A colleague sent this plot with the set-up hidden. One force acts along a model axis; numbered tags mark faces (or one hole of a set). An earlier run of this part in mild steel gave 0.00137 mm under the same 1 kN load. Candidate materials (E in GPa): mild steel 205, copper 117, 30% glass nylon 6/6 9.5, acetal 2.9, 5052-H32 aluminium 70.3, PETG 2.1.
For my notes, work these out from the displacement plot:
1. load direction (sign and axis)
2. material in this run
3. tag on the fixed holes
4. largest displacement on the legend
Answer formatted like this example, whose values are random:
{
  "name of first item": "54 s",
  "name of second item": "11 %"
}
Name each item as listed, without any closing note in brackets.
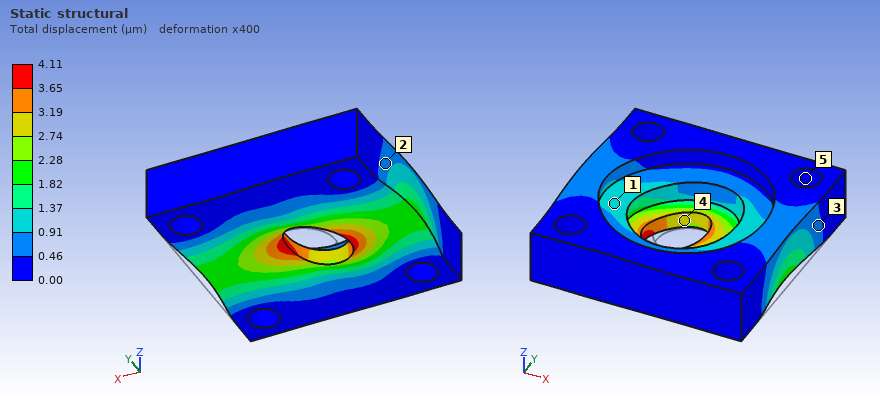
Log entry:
{
  "load direction": "-X",
  "material in this run": "5052-H32 aluminium",
  "tag on the fixed holes": "5",
  "largest displacement on the legend": "4.11 µm"
}
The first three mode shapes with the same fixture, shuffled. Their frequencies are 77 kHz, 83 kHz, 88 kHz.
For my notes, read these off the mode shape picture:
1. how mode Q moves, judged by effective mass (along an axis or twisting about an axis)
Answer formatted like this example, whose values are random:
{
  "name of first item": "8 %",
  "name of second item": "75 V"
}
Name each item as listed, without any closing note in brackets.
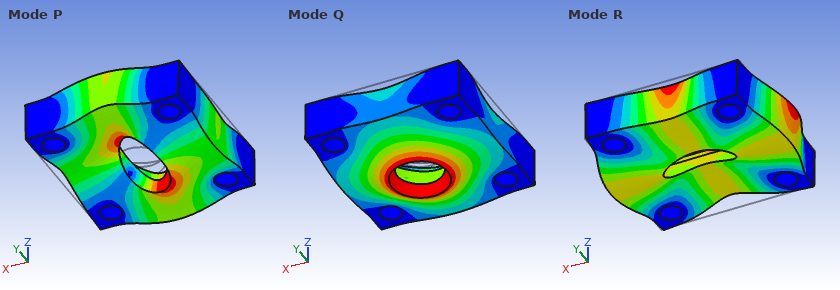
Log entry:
{
  "how mode Q moves, judged by effective mass": "along Z"
}
